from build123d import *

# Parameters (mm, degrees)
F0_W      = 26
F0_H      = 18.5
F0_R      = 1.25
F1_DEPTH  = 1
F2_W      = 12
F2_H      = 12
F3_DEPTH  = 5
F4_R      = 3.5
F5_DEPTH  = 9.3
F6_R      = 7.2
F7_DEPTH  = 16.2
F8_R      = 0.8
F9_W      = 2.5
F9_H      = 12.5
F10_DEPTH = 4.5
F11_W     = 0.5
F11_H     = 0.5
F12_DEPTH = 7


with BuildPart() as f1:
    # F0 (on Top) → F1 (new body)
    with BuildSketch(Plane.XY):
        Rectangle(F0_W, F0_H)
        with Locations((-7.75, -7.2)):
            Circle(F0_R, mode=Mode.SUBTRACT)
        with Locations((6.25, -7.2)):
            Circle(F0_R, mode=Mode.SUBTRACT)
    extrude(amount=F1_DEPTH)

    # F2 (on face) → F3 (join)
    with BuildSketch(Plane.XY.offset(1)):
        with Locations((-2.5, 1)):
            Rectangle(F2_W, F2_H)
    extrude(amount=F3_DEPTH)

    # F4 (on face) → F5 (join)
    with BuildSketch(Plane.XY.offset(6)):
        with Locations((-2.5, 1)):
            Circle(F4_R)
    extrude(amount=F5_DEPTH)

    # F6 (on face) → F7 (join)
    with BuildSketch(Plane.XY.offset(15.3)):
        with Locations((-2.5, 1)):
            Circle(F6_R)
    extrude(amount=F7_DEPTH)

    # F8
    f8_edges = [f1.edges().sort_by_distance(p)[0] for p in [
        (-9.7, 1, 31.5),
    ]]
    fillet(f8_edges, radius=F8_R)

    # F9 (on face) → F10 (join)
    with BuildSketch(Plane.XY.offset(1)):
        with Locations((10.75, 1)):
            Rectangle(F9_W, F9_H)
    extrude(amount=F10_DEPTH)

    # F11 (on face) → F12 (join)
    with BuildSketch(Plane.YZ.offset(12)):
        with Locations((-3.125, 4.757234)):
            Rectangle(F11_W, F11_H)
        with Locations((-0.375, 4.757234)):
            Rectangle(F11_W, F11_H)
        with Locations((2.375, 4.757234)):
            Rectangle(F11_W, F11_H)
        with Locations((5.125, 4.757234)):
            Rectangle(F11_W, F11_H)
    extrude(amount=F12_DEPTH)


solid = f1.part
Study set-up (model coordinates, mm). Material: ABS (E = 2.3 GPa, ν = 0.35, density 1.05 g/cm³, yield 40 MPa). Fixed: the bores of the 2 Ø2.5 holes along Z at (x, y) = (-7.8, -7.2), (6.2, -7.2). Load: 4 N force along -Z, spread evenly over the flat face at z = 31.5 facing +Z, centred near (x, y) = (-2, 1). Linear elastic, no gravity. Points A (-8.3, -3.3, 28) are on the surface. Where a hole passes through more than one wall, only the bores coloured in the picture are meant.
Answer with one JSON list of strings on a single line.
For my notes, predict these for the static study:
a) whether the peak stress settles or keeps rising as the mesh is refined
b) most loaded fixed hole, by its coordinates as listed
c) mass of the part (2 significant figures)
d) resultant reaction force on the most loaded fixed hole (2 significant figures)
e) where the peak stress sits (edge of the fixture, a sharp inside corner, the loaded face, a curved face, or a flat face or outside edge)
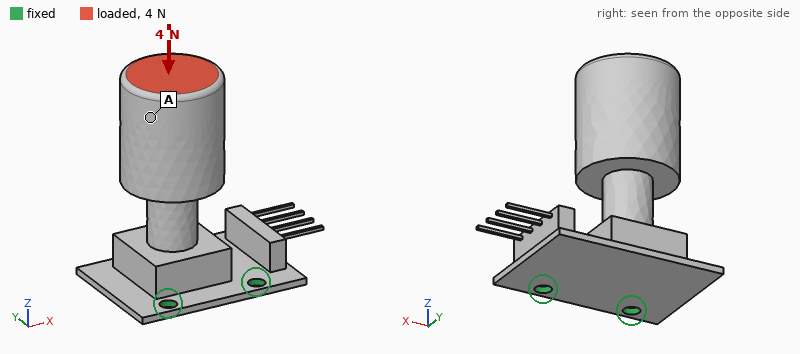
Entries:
["keeps rising", "(-7.8, -7.2)", "4.5 g", "2.3 N", "edge of the fixture"]
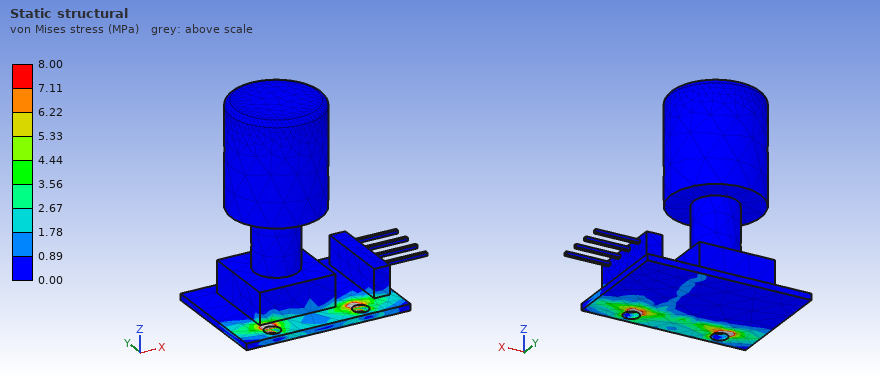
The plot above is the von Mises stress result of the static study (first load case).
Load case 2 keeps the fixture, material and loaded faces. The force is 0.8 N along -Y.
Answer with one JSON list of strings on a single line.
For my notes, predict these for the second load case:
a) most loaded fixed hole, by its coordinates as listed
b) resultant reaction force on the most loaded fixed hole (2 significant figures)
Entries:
["(-7.8, -7.2)", "0.63 N"]
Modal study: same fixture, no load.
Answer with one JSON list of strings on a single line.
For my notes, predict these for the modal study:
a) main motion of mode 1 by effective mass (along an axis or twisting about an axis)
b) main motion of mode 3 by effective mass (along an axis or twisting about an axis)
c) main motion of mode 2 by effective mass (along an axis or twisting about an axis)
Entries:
["along Y", "along Z", "along X"]
